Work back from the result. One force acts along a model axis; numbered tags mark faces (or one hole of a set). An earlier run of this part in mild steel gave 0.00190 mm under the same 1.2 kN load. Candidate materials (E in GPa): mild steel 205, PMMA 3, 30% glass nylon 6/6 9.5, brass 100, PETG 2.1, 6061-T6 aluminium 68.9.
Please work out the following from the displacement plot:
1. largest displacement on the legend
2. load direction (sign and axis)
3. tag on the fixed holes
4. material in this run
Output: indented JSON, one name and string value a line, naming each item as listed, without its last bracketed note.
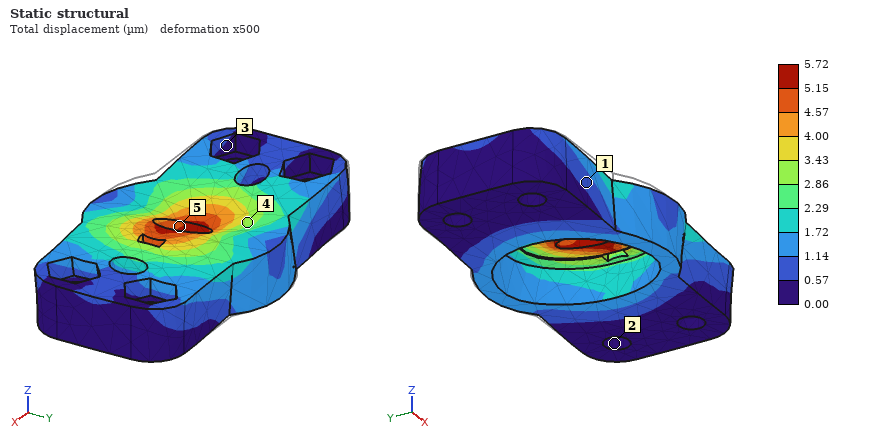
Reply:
{
  "largest displacement on the legend": "5.72 µm",
  "load direction": "+X",
  "tag on the fixed holes": "2",
  "material in this run": "6061-T6 aluminium"
}
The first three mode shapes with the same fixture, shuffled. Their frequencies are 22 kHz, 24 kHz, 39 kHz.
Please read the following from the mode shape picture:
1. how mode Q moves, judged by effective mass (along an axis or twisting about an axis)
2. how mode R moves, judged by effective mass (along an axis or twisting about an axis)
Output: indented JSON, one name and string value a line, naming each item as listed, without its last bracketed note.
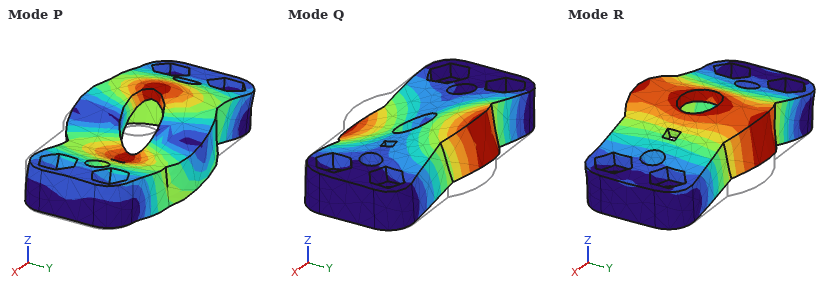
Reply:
{
  "how mode Q moves, judged by effective mass": "twisting about X",
  "how mode R moves, judged by effective mass": "along Z"
}
